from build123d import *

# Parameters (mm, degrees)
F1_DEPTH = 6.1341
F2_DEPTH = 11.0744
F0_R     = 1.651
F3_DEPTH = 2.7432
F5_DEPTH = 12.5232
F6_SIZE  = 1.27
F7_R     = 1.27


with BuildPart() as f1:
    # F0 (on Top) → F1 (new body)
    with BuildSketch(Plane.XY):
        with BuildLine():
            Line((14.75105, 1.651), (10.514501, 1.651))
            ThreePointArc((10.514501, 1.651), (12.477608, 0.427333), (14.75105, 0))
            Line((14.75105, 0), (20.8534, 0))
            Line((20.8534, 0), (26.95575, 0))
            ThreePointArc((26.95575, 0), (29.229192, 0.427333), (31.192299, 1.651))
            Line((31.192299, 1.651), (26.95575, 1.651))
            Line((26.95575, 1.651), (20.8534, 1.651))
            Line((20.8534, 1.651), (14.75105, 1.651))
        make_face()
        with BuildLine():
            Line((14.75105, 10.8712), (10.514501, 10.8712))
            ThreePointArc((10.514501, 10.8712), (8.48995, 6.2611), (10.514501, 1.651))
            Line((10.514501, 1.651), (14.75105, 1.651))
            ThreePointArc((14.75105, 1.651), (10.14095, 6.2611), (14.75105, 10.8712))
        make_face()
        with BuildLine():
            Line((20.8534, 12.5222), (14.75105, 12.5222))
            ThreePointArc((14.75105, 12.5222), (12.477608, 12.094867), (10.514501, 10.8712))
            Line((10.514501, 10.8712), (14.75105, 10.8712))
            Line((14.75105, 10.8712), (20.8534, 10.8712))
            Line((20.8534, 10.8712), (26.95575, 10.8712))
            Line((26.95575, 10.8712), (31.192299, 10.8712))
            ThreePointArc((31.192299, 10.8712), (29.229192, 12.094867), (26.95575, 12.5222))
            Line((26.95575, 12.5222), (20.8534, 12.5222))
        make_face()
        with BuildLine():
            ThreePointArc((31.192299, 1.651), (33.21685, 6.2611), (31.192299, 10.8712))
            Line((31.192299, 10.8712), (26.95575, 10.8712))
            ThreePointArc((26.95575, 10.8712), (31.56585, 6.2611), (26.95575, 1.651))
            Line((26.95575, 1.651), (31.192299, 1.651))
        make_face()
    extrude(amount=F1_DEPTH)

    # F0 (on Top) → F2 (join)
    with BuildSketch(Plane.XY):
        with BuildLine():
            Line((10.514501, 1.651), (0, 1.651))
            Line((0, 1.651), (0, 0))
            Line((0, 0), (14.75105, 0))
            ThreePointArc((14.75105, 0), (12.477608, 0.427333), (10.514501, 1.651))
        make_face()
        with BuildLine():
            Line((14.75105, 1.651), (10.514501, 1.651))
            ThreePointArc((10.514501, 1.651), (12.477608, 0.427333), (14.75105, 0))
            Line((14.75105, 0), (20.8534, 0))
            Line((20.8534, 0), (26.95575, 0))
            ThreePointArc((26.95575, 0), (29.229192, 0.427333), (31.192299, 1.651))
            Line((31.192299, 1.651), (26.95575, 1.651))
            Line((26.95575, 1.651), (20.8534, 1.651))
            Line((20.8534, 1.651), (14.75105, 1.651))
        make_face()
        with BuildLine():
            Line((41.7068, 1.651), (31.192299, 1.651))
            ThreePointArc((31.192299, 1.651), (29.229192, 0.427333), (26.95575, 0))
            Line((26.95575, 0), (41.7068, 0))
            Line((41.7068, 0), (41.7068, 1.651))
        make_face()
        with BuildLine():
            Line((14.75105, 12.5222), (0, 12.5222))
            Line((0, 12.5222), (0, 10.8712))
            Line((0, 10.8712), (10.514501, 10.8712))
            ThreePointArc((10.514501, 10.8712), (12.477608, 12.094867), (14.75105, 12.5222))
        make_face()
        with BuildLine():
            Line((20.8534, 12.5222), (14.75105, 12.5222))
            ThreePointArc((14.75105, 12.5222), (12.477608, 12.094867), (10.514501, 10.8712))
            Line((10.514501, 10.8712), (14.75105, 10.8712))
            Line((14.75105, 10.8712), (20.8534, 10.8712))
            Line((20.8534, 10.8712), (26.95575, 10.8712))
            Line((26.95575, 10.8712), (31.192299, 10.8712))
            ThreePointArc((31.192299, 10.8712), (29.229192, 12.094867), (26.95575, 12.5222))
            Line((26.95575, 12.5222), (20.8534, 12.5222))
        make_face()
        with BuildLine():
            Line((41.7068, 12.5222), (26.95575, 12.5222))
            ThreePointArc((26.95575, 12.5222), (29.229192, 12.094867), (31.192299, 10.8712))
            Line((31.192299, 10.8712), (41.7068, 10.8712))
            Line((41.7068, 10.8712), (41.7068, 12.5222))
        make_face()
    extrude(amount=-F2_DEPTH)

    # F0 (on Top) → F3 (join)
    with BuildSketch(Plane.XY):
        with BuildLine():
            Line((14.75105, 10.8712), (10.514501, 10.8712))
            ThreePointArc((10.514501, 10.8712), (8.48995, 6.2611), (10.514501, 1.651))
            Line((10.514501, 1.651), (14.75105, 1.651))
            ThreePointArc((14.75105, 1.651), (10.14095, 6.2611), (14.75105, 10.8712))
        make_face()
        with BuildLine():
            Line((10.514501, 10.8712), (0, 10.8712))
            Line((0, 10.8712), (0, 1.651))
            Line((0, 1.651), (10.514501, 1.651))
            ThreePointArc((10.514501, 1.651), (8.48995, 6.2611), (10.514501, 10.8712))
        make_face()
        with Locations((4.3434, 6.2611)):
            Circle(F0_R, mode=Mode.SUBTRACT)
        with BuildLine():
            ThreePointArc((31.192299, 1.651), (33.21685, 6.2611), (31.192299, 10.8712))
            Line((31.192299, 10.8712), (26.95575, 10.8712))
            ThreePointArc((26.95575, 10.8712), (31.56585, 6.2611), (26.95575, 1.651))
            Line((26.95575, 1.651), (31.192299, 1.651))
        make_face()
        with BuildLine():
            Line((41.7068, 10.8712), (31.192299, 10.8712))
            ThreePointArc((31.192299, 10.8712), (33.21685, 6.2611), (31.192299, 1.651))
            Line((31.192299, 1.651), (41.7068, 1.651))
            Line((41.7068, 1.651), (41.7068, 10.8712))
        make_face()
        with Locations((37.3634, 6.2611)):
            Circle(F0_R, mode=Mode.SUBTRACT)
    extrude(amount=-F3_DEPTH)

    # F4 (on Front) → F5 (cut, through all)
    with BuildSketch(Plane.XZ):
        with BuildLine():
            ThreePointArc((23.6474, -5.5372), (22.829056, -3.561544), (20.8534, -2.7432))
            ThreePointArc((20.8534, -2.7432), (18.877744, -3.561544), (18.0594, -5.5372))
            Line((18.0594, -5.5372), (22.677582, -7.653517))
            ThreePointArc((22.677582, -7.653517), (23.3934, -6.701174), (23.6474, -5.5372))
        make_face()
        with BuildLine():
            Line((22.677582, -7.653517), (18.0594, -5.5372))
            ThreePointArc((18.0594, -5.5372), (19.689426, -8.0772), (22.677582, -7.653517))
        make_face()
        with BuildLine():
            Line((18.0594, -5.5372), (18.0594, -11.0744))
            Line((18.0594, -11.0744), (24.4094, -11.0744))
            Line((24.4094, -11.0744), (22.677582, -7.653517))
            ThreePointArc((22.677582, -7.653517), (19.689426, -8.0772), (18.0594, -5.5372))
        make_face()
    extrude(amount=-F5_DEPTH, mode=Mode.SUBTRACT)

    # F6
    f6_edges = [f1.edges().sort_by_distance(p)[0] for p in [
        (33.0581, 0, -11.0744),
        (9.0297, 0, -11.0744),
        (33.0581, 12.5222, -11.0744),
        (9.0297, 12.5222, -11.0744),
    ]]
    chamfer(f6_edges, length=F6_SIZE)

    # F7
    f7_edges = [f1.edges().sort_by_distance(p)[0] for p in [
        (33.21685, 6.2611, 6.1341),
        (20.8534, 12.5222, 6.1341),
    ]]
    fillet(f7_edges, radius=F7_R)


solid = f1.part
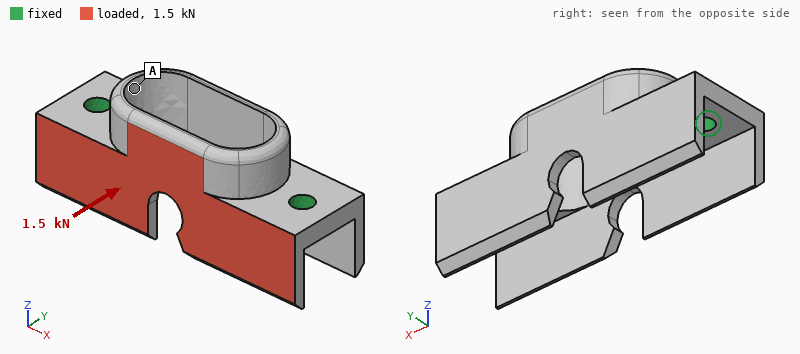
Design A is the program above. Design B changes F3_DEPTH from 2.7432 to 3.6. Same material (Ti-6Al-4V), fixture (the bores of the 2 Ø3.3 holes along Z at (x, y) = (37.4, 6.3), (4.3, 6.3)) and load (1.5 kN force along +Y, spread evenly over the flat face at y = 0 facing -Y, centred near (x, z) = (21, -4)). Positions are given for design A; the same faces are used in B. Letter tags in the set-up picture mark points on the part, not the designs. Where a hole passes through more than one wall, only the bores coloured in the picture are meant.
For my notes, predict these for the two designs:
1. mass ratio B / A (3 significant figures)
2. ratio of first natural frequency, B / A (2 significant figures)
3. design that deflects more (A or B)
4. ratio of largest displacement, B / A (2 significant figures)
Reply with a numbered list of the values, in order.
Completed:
1. 1.07
2. 1.3
3. A
4. 0.69
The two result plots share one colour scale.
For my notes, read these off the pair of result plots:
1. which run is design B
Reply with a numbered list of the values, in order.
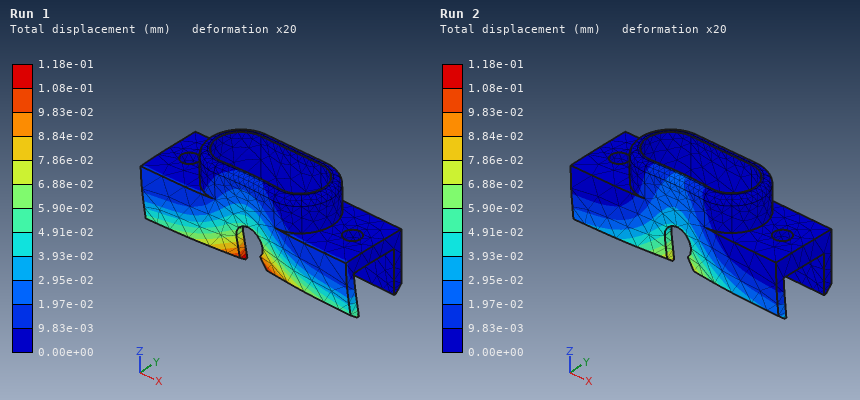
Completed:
1. Run 2
